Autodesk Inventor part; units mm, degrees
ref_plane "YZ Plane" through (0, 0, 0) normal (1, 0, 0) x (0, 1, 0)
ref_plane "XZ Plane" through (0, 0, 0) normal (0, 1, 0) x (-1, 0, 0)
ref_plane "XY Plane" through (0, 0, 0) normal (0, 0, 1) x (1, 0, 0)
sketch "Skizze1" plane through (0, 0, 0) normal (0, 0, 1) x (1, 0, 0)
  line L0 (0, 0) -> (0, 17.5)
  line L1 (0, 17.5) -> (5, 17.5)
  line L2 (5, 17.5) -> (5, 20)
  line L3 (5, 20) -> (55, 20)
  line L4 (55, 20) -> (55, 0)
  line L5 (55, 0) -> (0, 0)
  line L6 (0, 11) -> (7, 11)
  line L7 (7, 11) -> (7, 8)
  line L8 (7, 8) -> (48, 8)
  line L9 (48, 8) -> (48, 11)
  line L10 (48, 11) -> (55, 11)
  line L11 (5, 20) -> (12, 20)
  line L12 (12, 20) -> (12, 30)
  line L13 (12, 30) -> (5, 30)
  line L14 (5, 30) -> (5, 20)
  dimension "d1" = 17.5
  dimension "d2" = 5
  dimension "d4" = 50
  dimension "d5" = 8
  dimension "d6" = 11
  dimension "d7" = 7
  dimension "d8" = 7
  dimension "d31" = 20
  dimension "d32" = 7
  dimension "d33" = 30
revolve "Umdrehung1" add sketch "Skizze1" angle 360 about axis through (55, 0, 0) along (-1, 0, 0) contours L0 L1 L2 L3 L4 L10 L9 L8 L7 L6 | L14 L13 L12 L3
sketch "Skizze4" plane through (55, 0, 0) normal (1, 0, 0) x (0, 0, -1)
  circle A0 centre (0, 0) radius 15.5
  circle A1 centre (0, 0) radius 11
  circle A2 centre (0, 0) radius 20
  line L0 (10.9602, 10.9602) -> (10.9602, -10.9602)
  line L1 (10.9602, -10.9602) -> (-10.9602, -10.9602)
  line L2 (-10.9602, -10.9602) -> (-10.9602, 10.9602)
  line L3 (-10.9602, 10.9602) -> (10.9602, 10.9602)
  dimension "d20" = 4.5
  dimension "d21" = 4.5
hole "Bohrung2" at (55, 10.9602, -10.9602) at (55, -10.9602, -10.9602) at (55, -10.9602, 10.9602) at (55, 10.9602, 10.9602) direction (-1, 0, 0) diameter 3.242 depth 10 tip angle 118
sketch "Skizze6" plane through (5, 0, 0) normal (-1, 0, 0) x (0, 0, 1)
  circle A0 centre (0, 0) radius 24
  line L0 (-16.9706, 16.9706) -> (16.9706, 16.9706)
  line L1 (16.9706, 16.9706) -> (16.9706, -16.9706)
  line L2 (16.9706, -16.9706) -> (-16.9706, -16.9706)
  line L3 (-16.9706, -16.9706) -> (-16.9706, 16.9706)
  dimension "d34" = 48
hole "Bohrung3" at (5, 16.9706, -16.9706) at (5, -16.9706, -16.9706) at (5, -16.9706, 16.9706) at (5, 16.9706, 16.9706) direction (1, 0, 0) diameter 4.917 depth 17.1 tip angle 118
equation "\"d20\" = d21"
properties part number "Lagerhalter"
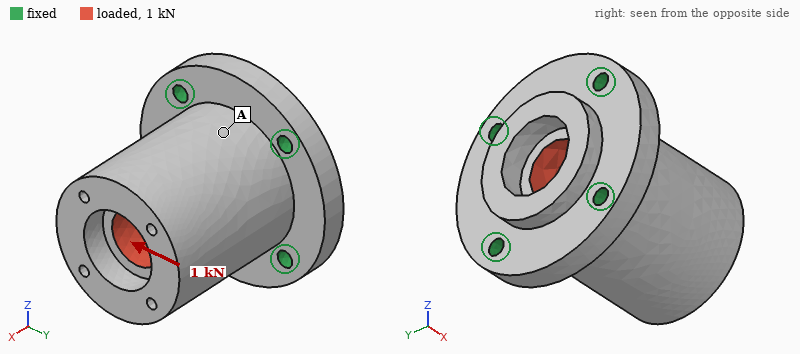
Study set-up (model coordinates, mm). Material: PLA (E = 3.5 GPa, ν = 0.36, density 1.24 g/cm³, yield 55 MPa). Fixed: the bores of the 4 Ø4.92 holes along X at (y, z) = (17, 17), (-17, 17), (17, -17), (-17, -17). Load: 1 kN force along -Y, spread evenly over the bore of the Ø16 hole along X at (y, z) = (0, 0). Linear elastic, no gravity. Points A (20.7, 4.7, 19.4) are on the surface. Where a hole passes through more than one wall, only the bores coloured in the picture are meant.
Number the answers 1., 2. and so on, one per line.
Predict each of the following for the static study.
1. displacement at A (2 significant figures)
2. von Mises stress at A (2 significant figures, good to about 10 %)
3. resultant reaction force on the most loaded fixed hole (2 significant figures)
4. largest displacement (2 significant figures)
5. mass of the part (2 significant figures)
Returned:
1. 24 µm
2. 1.5 MPa
3. 390 N
4. 87 µm
5. 80 g
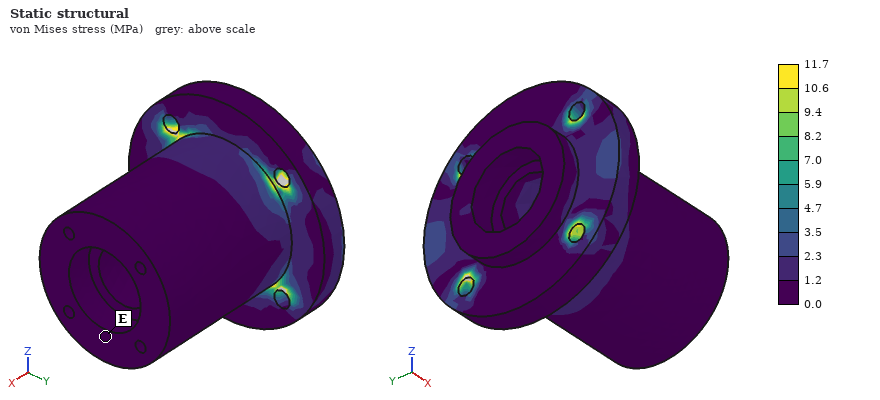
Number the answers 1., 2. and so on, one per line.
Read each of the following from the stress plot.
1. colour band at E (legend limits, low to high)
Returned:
1. 0.0 to 1.2 MPa
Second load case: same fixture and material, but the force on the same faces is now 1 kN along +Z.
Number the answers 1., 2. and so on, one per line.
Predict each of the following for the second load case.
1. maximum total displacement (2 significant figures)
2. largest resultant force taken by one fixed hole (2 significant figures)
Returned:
1. 87 µm
2. 390 N
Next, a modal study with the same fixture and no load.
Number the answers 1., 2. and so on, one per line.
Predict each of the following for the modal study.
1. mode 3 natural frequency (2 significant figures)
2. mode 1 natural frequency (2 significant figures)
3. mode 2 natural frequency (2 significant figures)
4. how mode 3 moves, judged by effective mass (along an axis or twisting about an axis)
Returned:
1. 4600 Hz
2. 2400 Hz
3. 2400 Hz
4. along X
